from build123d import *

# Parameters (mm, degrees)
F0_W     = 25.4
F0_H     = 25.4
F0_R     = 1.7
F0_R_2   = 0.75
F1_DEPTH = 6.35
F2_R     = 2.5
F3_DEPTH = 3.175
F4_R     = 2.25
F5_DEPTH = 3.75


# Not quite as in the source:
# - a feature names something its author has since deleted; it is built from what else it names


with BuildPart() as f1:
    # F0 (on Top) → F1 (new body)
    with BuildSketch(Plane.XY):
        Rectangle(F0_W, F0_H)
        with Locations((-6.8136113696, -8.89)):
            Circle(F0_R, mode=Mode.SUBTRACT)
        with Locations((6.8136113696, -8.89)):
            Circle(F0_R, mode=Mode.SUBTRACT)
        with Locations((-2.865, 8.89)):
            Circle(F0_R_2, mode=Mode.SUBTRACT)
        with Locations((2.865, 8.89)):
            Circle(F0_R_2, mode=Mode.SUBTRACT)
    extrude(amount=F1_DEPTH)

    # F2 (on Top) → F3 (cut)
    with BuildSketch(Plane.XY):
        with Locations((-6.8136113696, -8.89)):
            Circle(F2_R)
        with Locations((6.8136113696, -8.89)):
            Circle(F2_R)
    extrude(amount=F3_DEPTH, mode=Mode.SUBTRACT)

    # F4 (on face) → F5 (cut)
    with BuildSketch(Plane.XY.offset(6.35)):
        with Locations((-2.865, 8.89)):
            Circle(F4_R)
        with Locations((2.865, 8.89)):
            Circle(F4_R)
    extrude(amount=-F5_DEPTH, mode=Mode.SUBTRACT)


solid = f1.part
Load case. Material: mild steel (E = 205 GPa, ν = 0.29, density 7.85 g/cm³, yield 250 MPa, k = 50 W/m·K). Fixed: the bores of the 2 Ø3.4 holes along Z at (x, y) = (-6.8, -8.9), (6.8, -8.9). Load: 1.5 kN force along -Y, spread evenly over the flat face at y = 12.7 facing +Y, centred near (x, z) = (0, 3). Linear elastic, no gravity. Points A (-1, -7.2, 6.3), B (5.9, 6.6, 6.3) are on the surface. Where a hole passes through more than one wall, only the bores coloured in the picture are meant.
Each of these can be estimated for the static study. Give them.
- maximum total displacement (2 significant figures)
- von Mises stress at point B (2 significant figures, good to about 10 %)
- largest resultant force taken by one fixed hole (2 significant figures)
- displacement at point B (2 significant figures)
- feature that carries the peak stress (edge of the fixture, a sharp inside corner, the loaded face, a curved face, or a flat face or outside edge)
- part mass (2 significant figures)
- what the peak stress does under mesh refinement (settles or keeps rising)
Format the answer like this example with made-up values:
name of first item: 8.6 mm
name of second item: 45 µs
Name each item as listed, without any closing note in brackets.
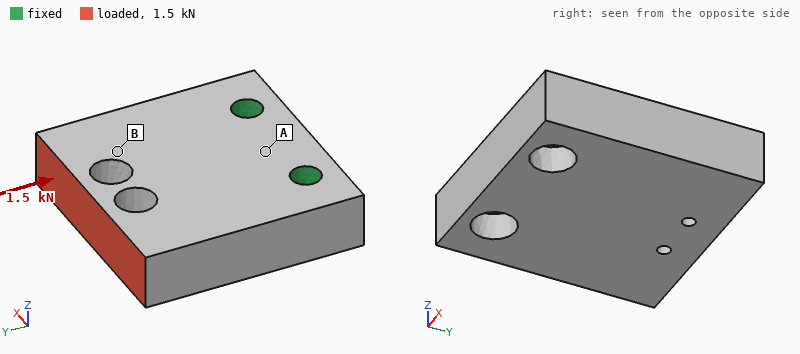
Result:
maximum total displacement: 5.1 µm
von Mises stress at point B: 17 MPa
largest resultant force taken by one fixed hole: 750 N
displacement at point B: 3.3 µm
feature that carries the peak stress: edge of the fixture
part mass: 30 g
what the peak stress does under mesh refinement: keeps rising
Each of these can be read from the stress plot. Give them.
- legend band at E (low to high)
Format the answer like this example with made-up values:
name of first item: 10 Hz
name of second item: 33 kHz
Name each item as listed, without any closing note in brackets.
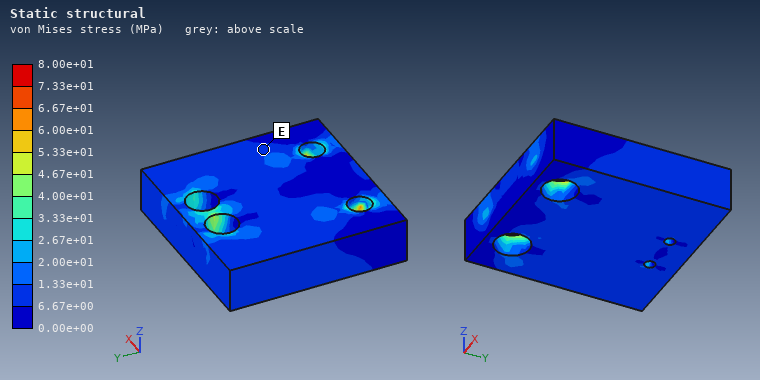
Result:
legend band at E: 6.67e+00 to 1.33e+01 MPa
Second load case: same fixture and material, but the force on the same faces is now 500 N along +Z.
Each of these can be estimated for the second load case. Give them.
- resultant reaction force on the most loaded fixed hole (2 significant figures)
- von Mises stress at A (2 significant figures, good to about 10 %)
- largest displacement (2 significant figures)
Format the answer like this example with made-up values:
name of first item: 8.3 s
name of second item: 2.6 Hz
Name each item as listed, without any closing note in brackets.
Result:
resultant reaction force on the most loaded fixed hole: 260 N
von Mises stress at A: 42 MPa
largest displacement: 33 µm
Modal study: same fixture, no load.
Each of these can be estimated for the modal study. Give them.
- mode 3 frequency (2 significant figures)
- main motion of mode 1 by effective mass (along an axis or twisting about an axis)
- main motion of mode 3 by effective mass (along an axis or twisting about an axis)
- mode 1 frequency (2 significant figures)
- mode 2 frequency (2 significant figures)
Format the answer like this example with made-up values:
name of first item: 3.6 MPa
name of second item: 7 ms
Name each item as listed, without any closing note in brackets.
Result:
mode 3 frequency: 21 kHz
main motion of mode 1 by effective mass: along Z
main motion of mode 3 by effective mass: along X
mode 1 frequency: 7300 Hz
mode 2 frequency: 17 kHz
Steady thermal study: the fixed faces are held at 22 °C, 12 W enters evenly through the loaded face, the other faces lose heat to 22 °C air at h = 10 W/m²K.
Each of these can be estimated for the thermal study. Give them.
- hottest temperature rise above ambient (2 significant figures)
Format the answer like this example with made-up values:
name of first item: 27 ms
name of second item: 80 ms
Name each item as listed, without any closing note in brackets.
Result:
hottest temperature rise above ambient: 40 K
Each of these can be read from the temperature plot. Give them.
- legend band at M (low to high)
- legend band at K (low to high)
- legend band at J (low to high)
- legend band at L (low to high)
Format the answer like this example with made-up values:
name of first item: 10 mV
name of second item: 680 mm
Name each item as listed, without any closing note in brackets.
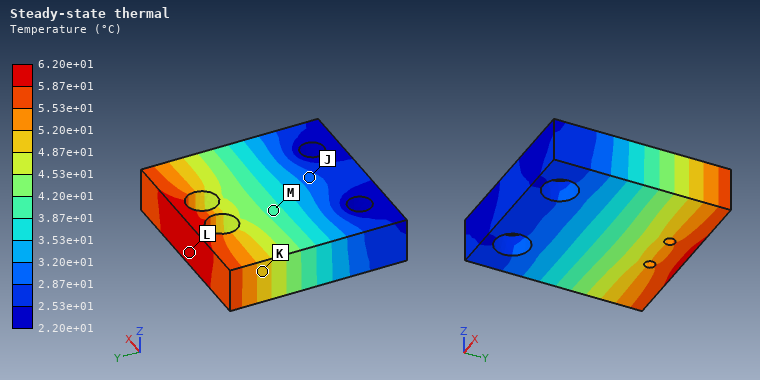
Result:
legend band at M: 3.87e+01 to 4.20e+01 °C
legend band at K: 4.87e+01 to 5.20e+01 °C
legend band at J: 2.87e+01 to 3.20e+01 °C
legend band at L: 5.87e+01 to 6.20e+01 °C
